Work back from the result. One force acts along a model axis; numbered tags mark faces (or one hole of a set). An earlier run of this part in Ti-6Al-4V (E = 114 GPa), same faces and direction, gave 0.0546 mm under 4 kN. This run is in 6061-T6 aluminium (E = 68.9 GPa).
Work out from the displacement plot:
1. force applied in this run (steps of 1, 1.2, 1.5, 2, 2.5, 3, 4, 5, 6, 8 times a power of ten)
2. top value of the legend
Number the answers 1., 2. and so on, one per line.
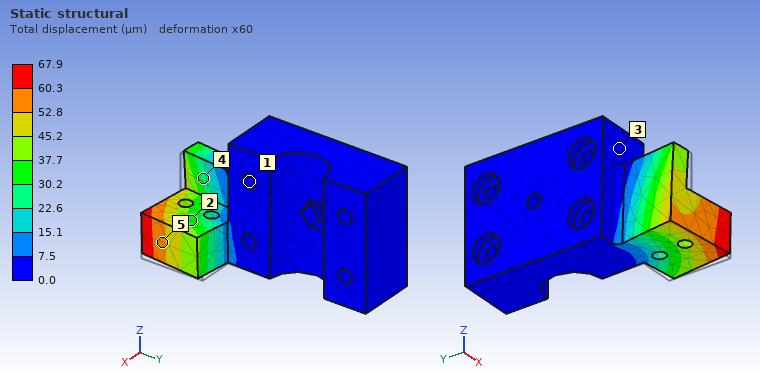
1. 3 kN
2. 67.9 µm
